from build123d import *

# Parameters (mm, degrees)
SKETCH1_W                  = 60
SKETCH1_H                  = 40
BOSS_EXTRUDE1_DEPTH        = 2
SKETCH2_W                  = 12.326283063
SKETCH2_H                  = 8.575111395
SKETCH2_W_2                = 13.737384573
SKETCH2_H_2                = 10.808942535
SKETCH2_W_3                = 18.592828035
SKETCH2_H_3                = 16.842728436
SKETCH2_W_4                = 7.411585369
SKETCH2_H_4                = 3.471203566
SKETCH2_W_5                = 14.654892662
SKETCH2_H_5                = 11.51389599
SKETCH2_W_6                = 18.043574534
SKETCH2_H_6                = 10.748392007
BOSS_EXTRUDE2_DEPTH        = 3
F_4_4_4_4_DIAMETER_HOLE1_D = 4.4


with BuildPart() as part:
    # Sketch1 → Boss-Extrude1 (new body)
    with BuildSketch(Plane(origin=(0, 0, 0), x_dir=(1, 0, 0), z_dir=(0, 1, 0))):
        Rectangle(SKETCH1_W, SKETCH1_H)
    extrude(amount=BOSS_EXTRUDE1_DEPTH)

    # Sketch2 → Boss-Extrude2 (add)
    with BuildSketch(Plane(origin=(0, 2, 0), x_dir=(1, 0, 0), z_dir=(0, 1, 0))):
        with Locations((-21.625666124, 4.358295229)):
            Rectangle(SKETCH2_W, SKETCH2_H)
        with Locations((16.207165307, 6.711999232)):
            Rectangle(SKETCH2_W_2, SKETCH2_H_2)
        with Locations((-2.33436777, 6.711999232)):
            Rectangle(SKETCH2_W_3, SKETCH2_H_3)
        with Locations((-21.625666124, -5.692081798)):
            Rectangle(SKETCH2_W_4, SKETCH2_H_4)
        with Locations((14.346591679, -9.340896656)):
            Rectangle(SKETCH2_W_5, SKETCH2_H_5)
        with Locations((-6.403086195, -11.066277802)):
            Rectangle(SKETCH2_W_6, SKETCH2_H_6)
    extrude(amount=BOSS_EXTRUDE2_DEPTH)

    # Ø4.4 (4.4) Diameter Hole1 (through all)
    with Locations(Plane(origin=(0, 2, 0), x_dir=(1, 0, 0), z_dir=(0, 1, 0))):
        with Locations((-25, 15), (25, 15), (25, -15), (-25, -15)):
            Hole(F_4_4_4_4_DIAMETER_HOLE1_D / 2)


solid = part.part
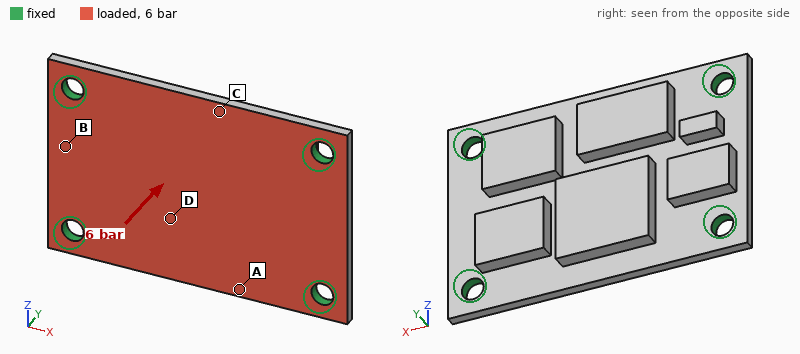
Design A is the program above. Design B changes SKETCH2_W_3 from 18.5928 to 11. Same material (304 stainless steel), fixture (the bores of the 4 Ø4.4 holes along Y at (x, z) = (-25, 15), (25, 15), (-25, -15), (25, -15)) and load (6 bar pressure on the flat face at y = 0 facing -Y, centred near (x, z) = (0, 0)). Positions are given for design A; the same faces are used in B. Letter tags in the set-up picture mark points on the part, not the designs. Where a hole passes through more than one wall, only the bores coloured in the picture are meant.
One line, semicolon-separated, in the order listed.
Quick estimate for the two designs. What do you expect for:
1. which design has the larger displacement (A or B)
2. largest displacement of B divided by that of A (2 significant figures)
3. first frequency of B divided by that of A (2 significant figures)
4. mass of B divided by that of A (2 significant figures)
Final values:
B; 1.2; 0.95; 0.95
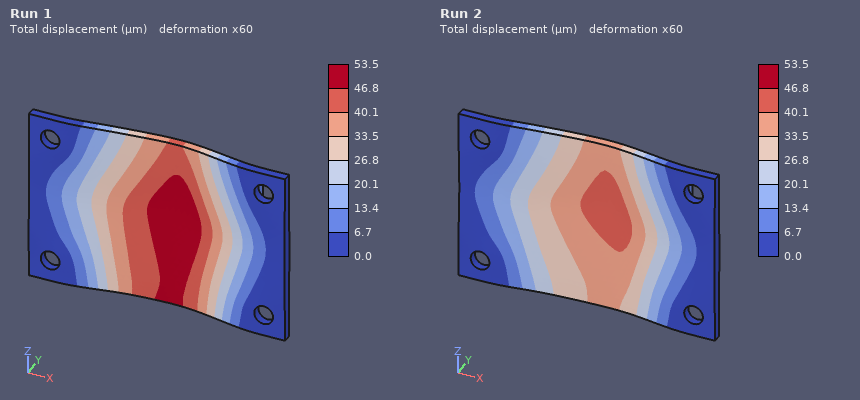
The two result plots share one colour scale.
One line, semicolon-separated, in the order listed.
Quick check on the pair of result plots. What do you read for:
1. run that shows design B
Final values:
Run 1
